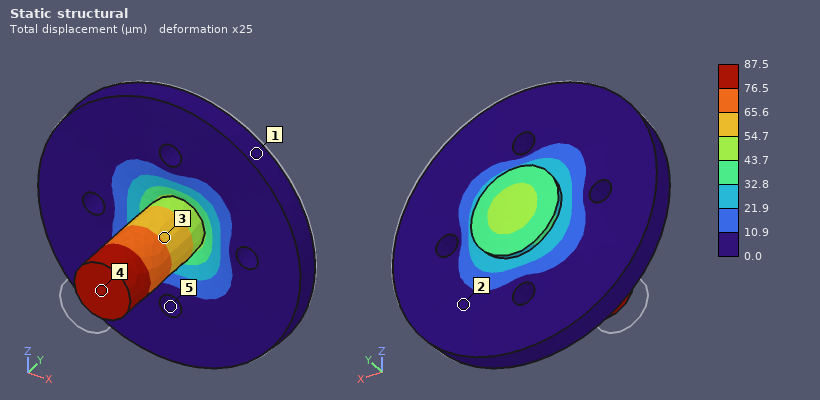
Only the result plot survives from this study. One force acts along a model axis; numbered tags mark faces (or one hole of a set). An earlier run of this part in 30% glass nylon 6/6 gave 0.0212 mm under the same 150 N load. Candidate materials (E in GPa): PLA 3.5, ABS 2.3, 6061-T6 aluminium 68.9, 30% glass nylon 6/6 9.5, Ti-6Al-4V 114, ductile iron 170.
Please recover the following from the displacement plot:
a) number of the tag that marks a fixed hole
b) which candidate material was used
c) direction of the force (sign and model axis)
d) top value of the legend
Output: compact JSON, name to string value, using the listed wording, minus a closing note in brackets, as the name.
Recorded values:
{"number of the tag that marks a fixed hole": "5", "which candidate material was used": "ABS", "direction of the force": "+Y", "top value of the legend": "87.5 µm"}
